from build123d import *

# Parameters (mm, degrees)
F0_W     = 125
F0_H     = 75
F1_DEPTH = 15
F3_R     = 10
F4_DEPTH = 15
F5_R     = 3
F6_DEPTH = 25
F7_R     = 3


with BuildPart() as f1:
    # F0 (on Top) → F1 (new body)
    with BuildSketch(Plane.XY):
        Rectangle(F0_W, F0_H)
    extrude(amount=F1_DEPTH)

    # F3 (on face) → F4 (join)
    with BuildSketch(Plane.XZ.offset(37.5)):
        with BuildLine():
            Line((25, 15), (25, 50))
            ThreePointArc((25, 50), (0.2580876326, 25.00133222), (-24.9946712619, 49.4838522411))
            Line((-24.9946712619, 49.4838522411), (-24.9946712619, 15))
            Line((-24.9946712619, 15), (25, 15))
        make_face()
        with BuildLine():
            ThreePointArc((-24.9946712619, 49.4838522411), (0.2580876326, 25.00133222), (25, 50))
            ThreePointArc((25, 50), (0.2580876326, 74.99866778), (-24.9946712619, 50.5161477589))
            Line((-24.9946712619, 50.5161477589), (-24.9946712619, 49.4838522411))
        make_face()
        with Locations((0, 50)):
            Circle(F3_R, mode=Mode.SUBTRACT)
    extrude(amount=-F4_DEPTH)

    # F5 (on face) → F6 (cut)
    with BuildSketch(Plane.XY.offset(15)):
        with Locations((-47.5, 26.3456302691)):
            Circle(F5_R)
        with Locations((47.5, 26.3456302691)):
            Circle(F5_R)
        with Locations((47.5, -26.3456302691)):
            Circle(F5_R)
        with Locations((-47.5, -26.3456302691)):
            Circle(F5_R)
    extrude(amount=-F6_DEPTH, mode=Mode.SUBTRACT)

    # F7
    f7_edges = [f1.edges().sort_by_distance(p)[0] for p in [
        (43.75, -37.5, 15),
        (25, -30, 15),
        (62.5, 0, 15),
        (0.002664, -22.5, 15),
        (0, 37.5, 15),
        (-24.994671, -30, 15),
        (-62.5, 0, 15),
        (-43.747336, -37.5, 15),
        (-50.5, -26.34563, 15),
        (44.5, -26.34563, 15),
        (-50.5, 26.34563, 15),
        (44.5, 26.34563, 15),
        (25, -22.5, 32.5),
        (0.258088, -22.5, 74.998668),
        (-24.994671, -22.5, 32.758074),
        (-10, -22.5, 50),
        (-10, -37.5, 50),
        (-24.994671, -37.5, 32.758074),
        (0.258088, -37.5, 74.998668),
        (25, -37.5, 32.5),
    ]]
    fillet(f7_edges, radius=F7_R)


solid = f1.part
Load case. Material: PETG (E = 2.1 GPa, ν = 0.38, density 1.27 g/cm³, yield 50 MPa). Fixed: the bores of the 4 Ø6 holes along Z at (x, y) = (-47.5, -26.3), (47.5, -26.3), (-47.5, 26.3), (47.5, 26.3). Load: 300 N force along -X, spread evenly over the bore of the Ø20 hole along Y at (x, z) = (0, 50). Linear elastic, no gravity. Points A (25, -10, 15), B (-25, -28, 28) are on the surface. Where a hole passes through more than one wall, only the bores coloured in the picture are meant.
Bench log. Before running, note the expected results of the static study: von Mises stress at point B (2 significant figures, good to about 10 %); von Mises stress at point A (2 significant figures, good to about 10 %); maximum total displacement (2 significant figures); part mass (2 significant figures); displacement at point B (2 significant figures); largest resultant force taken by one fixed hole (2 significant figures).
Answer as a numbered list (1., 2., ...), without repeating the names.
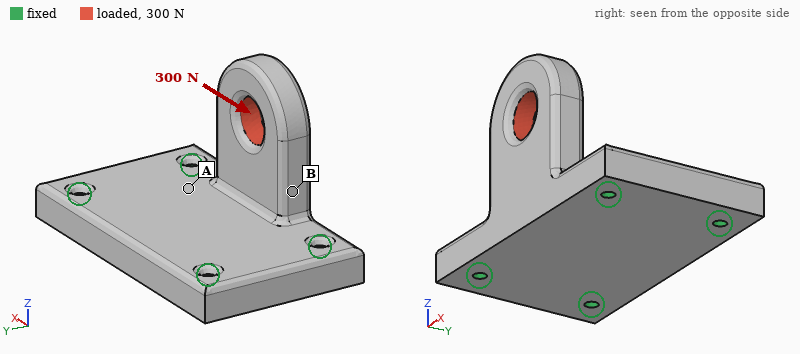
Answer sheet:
1. 1.5 MPa
2. 0.66 MPa
3. 0.15 mm
4. 220 g
5. 0.057 mm
6. 200 N
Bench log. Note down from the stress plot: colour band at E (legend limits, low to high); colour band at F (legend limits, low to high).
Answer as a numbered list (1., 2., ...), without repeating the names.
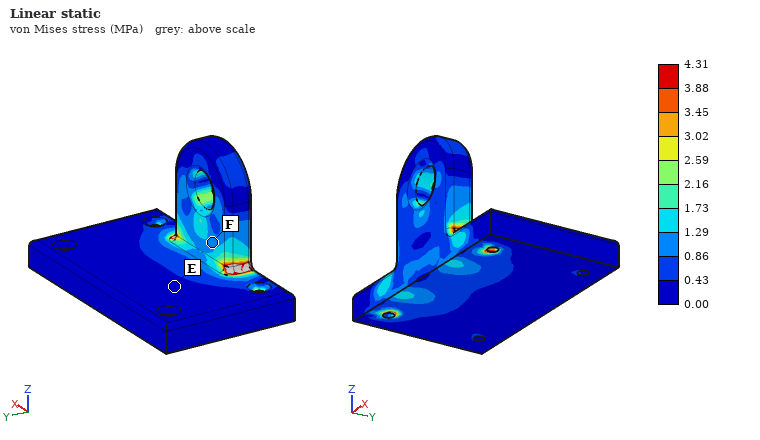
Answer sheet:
1. 0.00 to 0.43 MPa
2. 0.86 to 1.29 MPa
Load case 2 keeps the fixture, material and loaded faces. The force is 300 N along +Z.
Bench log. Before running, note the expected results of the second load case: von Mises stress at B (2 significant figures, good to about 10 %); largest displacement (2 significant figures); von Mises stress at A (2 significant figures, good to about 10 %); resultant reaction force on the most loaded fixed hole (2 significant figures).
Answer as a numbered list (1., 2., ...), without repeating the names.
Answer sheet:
1. 0.64 MPa
2. 0.11 mm
3. 0.61 MPa
4. 170 N
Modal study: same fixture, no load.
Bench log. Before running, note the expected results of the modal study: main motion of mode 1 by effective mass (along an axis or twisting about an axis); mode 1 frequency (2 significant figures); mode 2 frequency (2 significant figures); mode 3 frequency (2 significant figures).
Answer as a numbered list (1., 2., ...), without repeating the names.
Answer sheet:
1. along Y
2. 670 Hz
3. 1400 Hz
4. 1400 Hz
